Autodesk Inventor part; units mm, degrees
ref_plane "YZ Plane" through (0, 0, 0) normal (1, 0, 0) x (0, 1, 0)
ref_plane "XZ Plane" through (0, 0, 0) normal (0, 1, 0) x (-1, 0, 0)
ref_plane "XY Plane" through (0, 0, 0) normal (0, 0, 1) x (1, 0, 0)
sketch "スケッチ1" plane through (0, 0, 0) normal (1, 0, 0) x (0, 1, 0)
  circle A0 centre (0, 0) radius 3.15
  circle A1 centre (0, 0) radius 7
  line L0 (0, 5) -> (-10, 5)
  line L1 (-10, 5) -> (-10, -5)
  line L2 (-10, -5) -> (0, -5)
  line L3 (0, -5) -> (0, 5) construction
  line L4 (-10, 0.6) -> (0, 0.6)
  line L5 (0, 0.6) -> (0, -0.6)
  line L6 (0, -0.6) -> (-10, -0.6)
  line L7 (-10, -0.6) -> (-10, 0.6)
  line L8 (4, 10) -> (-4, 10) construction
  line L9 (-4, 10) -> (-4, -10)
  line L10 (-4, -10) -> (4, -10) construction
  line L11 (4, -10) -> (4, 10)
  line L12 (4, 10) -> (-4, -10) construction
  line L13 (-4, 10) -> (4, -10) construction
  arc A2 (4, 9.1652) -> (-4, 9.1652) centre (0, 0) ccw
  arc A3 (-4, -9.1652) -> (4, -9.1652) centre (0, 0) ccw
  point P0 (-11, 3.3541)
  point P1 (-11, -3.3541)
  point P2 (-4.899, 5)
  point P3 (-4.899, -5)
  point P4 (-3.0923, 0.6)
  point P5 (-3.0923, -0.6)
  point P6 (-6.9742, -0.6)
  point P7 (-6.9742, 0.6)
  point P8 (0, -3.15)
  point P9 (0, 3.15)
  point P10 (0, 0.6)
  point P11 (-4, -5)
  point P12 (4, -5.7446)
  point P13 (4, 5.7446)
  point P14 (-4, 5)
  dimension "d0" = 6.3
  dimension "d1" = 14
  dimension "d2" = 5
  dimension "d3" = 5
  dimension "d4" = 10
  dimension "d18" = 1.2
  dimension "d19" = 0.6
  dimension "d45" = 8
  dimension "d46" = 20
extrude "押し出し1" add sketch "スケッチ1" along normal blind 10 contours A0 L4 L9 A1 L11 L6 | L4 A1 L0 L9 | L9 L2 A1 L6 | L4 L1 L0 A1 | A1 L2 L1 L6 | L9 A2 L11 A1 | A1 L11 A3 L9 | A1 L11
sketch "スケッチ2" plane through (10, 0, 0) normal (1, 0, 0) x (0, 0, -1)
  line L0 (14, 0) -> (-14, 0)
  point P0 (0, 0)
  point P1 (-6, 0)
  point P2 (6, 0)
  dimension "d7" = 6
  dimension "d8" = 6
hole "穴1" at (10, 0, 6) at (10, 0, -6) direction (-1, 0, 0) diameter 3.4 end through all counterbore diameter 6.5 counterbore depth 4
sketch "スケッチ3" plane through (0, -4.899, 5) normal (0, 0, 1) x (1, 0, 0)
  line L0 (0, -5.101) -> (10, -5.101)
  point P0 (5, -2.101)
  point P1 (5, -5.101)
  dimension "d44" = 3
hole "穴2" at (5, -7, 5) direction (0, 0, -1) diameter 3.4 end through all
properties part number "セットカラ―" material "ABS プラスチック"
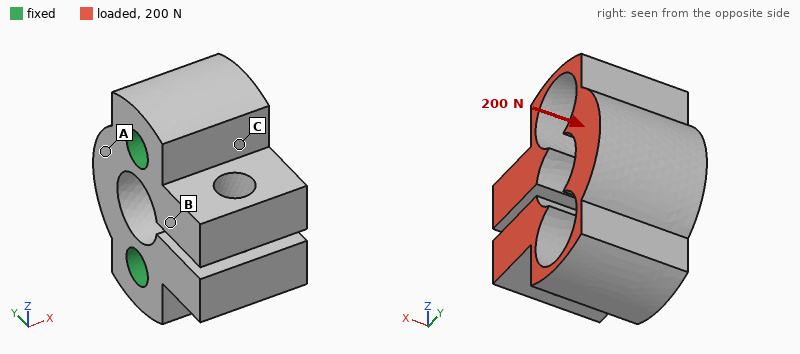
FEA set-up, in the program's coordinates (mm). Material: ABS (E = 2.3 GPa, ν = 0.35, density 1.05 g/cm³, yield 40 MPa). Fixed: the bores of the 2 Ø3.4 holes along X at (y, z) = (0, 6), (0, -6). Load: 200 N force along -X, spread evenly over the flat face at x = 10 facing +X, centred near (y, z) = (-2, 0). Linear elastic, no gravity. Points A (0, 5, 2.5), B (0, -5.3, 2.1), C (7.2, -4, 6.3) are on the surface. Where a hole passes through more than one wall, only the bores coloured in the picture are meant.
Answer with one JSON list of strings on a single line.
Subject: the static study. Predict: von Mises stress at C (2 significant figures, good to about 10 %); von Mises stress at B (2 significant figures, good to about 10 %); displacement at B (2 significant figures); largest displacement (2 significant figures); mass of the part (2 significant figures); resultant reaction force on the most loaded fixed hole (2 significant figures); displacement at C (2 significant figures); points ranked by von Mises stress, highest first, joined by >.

["4.5 MPa", "2.9 MPa", "29 µm", "79 µm", "1.6 g", "100 N", "16 µm", "C > B > A"]
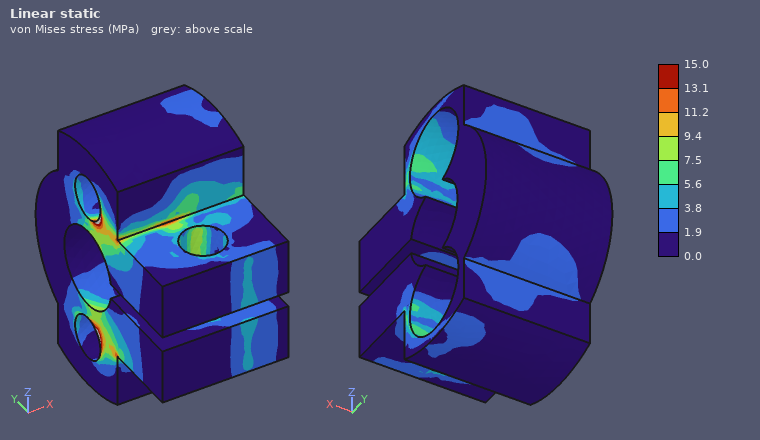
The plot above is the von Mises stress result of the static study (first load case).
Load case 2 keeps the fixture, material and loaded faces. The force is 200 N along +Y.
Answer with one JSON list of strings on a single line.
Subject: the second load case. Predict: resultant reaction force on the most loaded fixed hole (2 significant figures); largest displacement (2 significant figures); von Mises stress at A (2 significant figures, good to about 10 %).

["100 N", "0.16 mm", "2.6 MPa"]
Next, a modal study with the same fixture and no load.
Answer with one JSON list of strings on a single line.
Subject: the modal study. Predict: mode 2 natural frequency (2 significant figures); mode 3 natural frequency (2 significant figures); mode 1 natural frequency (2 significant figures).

["7300 Hz", "8700 Hz", "7300 Hz"]
